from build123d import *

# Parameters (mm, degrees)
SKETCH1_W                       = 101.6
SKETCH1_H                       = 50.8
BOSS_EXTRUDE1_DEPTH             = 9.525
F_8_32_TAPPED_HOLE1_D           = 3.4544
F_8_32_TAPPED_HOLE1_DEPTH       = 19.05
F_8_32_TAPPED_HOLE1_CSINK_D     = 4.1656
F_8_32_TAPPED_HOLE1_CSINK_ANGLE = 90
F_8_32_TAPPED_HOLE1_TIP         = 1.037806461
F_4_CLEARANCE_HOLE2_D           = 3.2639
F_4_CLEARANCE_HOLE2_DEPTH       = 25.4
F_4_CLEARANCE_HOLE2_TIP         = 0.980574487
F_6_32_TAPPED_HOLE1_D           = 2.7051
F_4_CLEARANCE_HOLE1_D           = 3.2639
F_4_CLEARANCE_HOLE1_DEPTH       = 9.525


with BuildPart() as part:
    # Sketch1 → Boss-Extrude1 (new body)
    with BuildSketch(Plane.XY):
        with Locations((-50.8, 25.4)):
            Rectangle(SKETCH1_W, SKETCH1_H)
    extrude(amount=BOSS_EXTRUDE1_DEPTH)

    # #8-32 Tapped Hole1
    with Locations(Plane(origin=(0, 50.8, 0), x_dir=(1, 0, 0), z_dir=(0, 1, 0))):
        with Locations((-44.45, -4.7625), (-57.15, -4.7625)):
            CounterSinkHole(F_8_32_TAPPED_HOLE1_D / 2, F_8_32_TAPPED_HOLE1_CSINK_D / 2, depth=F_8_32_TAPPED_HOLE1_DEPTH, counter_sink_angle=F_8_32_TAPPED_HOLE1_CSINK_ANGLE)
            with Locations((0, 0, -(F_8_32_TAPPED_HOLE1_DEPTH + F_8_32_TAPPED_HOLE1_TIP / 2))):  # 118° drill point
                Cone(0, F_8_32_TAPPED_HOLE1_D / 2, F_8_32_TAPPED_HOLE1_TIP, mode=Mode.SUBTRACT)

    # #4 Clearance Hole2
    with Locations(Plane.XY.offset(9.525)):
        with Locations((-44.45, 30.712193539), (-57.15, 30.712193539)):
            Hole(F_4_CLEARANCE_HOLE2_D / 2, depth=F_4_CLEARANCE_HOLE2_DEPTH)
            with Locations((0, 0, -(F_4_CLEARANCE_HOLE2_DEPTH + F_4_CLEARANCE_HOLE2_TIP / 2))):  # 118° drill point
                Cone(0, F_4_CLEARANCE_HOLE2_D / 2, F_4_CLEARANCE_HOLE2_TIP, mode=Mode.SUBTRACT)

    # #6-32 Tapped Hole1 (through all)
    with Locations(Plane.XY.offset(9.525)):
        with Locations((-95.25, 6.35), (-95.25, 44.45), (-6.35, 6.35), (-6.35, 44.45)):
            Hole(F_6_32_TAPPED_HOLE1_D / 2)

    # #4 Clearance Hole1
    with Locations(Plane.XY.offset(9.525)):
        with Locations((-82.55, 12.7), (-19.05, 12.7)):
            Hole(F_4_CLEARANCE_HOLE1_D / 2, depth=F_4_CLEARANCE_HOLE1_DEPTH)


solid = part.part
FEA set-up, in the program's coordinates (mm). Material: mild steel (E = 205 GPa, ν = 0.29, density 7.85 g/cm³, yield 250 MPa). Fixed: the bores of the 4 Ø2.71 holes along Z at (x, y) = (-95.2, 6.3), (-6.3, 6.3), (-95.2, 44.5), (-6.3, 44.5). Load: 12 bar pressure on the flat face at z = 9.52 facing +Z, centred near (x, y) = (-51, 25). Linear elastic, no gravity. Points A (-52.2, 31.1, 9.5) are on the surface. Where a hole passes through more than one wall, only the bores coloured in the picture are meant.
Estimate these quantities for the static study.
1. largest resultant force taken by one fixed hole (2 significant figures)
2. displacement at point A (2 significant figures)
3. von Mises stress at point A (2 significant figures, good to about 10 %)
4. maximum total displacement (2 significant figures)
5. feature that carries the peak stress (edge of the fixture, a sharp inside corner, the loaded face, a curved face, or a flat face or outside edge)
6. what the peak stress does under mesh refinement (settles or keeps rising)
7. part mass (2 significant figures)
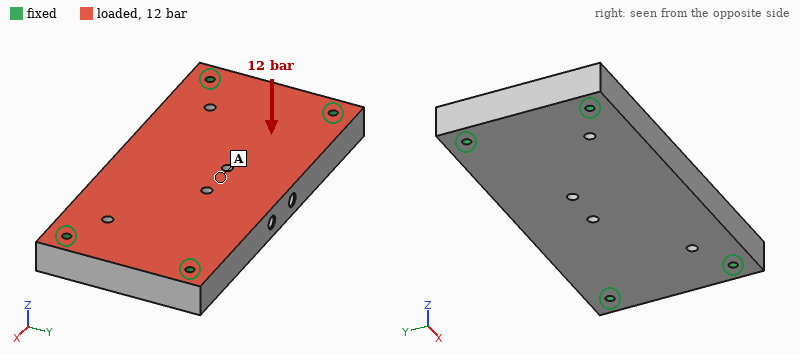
1.5 kN
22 µm
21 MPa
23 µm
edge of the fixture
keeps rising
380 g
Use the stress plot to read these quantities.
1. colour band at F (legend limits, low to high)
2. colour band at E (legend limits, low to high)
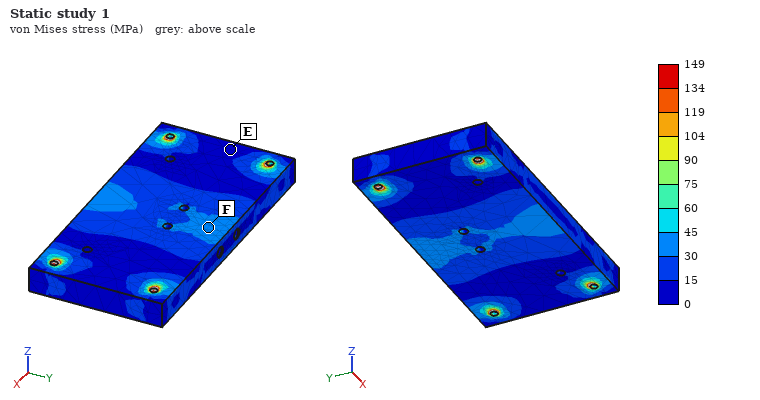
30 to 45 MPa
0 to 15 MPa
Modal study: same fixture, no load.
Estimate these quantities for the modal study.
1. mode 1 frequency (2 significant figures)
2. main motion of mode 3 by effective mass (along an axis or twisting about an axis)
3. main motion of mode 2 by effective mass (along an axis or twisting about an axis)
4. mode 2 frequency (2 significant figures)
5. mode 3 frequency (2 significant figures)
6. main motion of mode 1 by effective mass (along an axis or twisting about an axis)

4900 Hz
twisting about Y
twisting about X
8200 Hz
13 kHz
along Z
